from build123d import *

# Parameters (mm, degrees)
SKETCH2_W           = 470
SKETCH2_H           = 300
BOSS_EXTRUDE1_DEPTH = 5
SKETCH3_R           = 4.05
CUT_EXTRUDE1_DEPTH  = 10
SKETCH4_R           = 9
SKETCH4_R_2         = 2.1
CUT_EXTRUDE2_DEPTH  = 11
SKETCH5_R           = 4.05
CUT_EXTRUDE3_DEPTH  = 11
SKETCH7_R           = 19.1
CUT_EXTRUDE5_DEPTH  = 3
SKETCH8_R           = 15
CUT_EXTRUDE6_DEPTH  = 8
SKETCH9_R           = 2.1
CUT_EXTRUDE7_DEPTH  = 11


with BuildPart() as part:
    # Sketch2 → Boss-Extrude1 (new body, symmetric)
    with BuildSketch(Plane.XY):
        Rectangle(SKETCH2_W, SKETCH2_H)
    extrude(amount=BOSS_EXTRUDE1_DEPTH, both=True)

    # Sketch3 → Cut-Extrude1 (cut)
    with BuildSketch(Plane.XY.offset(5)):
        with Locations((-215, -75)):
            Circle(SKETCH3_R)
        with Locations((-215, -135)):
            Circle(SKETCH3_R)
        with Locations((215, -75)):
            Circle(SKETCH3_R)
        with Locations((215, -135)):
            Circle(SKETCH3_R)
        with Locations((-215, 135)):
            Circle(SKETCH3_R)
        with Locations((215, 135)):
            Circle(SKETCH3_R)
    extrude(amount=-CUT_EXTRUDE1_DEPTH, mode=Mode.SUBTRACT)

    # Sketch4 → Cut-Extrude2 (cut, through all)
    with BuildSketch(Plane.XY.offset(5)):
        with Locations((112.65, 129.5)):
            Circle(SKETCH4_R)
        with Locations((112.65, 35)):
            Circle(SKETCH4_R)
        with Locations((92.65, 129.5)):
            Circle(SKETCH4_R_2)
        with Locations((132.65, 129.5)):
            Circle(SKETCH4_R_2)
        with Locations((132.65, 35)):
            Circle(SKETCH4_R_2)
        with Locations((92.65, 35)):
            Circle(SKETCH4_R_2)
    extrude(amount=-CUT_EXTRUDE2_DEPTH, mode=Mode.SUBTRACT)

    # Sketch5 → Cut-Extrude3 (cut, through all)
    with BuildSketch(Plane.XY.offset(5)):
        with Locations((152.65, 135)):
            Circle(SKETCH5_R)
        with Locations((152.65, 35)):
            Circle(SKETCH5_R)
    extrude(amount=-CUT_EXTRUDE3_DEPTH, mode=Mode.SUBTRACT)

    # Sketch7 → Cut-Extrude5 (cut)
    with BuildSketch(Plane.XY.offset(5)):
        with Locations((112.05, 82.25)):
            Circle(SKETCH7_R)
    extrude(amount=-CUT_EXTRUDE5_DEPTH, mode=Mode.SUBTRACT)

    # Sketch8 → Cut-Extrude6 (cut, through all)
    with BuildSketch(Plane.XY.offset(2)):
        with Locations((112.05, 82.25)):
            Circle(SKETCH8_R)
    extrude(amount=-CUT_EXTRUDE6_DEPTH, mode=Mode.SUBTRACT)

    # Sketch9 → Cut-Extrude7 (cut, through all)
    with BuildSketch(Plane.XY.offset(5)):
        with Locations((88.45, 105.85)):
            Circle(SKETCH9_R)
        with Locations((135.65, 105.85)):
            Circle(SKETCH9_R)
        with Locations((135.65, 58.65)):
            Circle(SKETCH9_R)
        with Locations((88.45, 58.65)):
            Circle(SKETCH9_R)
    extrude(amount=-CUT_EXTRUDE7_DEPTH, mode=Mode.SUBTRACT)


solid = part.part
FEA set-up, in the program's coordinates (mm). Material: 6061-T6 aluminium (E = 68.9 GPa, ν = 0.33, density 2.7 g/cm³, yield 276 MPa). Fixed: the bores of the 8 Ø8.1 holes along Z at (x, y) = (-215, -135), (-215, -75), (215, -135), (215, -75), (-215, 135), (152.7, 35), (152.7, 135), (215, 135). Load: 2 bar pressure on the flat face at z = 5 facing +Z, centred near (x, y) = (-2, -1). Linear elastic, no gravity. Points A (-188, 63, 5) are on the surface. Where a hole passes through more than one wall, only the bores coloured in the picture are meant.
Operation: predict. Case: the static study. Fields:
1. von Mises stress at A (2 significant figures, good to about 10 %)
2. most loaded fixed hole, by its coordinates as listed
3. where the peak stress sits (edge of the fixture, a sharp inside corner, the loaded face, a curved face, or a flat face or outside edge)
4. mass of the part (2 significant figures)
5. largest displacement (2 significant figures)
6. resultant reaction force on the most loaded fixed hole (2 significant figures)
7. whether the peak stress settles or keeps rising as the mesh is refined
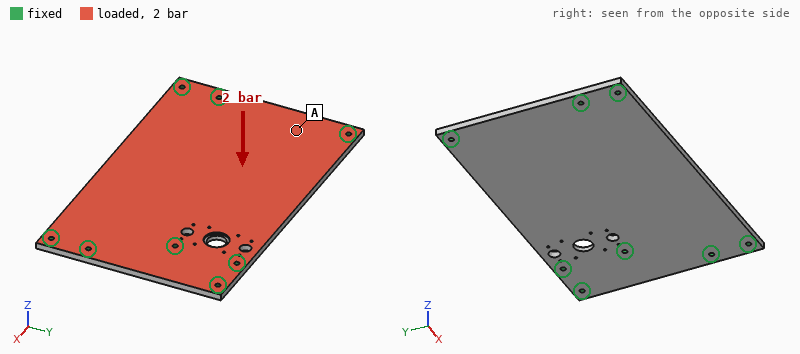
37 MPa
(152.7, 35)
edge of the fixture
3.8 kg
3.2 mm
8.6 kN
keeps rising
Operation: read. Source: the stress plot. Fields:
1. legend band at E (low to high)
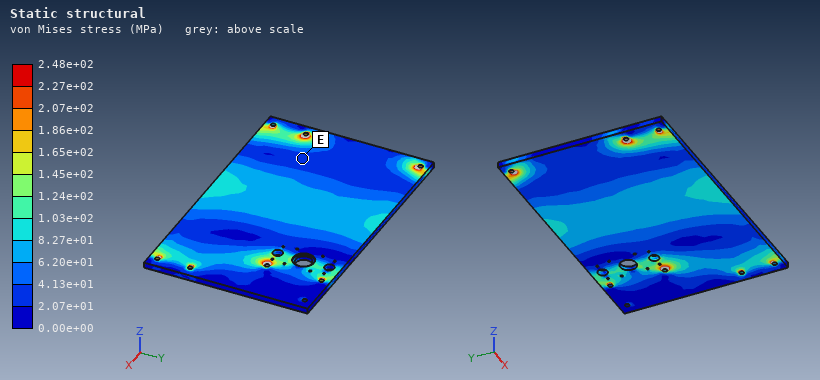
2.07e+01 to 4.13e+01 MPa
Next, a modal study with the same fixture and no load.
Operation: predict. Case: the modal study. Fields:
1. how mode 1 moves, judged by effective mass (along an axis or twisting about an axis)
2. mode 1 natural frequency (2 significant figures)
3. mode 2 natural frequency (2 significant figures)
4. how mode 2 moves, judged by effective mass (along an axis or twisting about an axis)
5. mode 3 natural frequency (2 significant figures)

along Z
300 Hz
420 Hz
twisting about X
790 Hz
